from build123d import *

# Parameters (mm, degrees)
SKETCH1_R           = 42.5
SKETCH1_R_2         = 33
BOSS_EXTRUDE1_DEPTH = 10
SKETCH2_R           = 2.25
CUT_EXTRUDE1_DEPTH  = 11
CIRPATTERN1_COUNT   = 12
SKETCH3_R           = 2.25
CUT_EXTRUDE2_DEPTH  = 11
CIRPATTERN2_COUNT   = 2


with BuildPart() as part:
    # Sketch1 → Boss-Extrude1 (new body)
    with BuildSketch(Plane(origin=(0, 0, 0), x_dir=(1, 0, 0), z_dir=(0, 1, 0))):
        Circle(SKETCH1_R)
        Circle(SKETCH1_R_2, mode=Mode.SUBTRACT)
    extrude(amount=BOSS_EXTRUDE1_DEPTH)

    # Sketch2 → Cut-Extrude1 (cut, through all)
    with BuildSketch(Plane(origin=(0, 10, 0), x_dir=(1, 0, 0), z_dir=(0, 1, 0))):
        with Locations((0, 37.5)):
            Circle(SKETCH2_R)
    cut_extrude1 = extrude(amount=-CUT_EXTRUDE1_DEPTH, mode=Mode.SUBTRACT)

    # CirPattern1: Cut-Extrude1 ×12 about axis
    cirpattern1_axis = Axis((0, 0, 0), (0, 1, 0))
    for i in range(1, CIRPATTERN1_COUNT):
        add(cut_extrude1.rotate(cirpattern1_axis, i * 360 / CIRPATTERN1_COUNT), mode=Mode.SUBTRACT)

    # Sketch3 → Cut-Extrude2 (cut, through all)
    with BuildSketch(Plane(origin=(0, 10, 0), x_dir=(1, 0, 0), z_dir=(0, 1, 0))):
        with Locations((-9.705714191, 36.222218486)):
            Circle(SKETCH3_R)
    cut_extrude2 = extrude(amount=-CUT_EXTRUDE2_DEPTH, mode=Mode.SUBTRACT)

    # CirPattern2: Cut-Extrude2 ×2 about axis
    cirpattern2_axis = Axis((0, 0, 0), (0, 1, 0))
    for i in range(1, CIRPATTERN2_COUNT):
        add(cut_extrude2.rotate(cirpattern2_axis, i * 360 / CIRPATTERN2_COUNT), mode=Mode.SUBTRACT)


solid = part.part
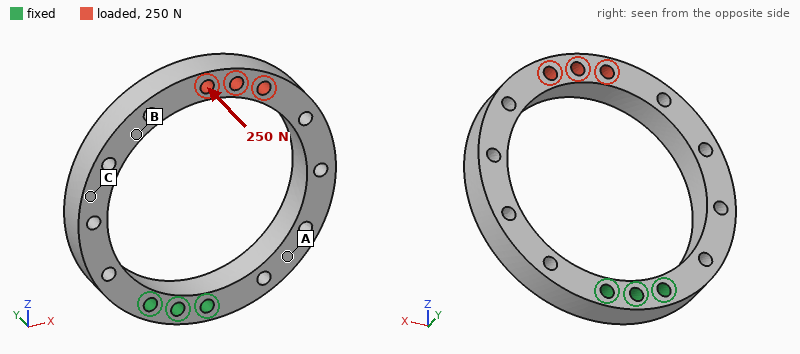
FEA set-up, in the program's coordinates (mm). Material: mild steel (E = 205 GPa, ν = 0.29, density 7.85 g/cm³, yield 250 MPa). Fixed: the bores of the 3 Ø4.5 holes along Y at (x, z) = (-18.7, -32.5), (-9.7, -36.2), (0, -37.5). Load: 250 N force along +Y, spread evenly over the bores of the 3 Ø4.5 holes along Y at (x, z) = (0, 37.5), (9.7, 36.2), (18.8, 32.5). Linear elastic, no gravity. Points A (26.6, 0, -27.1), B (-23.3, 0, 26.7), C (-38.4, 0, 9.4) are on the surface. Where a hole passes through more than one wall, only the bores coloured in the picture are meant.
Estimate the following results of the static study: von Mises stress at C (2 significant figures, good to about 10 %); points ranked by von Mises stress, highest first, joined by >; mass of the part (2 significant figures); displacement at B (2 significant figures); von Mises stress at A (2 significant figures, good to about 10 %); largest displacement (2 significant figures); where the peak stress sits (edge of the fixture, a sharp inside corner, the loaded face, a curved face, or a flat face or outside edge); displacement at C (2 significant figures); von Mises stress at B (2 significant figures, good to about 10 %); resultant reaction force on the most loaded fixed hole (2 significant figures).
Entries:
30 MPa
A > C > B
160 g
0.15 mm
50 MPa
0.25 mm
a curved face
0.072 mm
13 MPa
150 N
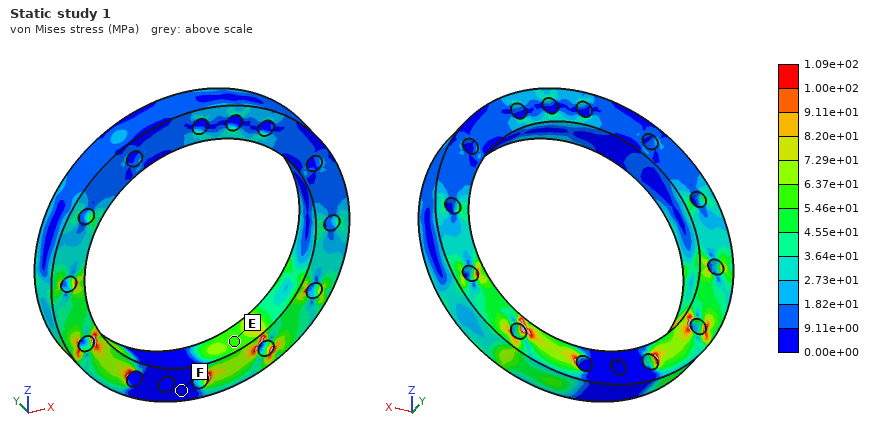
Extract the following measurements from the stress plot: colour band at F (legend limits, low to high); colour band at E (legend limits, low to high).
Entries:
0.00e+00 to 9.11e+00 MPa
5.46e+01 to 6.37e+01 MPa
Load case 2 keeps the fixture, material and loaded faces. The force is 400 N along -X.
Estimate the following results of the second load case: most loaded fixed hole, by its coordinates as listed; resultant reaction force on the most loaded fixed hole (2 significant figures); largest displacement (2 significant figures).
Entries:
(-18.7, -32.5)
620 N
0.11 mm
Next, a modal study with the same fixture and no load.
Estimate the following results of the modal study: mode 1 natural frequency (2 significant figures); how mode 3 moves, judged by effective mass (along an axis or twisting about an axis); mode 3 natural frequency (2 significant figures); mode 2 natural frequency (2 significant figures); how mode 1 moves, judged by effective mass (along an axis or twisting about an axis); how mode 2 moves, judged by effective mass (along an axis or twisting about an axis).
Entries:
740 Hz
twisting about Z
1800 Hz
1200 Hz
along Y
along X
